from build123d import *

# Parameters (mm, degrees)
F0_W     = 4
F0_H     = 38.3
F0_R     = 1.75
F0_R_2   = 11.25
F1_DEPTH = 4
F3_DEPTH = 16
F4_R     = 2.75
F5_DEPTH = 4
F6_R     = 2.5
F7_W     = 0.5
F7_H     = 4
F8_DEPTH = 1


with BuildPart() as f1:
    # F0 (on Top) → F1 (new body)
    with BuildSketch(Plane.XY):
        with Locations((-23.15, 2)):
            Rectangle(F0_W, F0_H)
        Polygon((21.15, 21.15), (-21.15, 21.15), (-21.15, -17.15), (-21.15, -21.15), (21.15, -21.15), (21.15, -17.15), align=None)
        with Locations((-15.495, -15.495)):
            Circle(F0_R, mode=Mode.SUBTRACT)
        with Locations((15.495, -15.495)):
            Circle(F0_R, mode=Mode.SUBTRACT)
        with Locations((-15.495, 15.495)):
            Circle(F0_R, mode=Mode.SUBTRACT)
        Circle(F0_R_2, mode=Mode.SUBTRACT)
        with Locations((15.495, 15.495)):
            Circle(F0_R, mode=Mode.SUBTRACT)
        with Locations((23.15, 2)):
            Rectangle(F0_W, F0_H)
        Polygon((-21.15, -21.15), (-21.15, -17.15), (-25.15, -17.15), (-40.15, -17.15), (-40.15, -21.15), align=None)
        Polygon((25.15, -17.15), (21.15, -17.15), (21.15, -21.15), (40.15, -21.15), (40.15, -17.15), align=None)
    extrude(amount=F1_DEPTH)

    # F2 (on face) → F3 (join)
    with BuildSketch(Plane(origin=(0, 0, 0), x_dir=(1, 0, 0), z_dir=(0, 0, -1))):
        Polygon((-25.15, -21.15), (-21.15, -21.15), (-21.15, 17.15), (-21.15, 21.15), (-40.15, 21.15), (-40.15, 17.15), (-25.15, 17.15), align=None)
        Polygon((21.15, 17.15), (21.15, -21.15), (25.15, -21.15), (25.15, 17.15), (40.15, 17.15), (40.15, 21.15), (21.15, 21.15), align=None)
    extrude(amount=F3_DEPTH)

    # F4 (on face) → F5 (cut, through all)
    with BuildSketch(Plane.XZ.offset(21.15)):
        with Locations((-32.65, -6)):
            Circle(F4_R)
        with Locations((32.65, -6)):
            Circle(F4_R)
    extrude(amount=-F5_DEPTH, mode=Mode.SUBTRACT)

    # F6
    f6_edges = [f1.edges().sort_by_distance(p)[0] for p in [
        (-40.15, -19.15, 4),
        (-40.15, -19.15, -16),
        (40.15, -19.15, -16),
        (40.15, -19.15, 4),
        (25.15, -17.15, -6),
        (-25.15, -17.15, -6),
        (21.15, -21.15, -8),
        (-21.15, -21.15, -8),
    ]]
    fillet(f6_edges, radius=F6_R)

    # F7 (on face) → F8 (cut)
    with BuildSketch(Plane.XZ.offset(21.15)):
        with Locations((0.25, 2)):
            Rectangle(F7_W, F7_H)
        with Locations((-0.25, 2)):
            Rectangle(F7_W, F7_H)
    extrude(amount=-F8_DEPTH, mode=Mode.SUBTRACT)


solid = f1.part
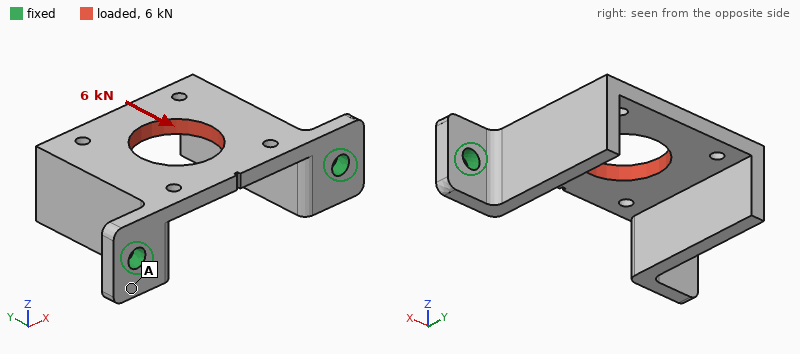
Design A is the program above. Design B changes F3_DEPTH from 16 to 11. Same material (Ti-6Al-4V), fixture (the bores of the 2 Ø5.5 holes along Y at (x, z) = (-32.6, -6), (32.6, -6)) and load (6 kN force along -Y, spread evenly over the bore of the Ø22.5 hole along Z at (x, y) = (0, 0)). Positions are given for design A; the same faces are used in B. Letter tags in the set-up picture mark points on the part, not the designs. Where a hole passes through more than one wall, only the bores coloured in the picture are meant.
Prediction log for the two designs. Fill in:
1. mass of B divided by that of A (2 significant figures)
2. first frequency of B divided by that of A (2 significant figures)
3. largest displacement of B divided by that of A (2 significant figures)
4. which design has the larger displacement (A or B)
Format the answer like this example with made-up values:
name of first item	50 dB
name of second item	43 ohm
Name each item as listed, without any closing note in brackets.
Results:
mass of B divided by that of A	0.84
first frequency of B divided by that of A	0.90
largest displacement of B divided by that of A	1.3
which design has the larger displacement	B
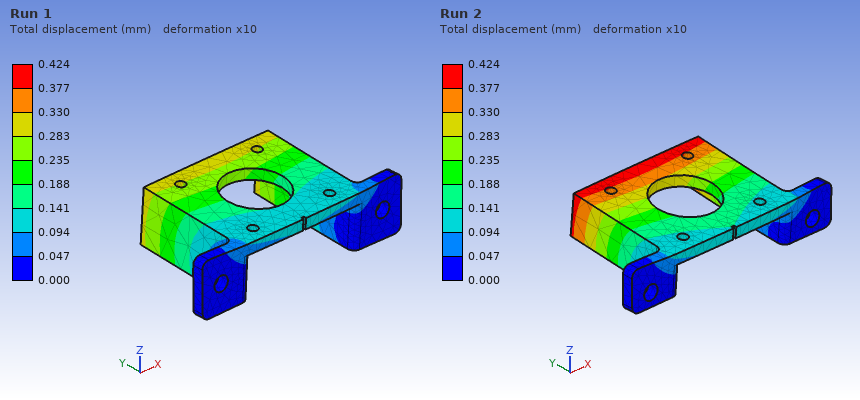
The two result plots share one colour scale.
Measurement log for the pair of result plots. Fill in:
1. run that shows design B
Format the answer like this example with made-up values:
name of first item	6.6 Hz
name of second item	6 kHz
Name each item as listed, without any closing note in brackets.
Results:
run that shows design B	Run 2
